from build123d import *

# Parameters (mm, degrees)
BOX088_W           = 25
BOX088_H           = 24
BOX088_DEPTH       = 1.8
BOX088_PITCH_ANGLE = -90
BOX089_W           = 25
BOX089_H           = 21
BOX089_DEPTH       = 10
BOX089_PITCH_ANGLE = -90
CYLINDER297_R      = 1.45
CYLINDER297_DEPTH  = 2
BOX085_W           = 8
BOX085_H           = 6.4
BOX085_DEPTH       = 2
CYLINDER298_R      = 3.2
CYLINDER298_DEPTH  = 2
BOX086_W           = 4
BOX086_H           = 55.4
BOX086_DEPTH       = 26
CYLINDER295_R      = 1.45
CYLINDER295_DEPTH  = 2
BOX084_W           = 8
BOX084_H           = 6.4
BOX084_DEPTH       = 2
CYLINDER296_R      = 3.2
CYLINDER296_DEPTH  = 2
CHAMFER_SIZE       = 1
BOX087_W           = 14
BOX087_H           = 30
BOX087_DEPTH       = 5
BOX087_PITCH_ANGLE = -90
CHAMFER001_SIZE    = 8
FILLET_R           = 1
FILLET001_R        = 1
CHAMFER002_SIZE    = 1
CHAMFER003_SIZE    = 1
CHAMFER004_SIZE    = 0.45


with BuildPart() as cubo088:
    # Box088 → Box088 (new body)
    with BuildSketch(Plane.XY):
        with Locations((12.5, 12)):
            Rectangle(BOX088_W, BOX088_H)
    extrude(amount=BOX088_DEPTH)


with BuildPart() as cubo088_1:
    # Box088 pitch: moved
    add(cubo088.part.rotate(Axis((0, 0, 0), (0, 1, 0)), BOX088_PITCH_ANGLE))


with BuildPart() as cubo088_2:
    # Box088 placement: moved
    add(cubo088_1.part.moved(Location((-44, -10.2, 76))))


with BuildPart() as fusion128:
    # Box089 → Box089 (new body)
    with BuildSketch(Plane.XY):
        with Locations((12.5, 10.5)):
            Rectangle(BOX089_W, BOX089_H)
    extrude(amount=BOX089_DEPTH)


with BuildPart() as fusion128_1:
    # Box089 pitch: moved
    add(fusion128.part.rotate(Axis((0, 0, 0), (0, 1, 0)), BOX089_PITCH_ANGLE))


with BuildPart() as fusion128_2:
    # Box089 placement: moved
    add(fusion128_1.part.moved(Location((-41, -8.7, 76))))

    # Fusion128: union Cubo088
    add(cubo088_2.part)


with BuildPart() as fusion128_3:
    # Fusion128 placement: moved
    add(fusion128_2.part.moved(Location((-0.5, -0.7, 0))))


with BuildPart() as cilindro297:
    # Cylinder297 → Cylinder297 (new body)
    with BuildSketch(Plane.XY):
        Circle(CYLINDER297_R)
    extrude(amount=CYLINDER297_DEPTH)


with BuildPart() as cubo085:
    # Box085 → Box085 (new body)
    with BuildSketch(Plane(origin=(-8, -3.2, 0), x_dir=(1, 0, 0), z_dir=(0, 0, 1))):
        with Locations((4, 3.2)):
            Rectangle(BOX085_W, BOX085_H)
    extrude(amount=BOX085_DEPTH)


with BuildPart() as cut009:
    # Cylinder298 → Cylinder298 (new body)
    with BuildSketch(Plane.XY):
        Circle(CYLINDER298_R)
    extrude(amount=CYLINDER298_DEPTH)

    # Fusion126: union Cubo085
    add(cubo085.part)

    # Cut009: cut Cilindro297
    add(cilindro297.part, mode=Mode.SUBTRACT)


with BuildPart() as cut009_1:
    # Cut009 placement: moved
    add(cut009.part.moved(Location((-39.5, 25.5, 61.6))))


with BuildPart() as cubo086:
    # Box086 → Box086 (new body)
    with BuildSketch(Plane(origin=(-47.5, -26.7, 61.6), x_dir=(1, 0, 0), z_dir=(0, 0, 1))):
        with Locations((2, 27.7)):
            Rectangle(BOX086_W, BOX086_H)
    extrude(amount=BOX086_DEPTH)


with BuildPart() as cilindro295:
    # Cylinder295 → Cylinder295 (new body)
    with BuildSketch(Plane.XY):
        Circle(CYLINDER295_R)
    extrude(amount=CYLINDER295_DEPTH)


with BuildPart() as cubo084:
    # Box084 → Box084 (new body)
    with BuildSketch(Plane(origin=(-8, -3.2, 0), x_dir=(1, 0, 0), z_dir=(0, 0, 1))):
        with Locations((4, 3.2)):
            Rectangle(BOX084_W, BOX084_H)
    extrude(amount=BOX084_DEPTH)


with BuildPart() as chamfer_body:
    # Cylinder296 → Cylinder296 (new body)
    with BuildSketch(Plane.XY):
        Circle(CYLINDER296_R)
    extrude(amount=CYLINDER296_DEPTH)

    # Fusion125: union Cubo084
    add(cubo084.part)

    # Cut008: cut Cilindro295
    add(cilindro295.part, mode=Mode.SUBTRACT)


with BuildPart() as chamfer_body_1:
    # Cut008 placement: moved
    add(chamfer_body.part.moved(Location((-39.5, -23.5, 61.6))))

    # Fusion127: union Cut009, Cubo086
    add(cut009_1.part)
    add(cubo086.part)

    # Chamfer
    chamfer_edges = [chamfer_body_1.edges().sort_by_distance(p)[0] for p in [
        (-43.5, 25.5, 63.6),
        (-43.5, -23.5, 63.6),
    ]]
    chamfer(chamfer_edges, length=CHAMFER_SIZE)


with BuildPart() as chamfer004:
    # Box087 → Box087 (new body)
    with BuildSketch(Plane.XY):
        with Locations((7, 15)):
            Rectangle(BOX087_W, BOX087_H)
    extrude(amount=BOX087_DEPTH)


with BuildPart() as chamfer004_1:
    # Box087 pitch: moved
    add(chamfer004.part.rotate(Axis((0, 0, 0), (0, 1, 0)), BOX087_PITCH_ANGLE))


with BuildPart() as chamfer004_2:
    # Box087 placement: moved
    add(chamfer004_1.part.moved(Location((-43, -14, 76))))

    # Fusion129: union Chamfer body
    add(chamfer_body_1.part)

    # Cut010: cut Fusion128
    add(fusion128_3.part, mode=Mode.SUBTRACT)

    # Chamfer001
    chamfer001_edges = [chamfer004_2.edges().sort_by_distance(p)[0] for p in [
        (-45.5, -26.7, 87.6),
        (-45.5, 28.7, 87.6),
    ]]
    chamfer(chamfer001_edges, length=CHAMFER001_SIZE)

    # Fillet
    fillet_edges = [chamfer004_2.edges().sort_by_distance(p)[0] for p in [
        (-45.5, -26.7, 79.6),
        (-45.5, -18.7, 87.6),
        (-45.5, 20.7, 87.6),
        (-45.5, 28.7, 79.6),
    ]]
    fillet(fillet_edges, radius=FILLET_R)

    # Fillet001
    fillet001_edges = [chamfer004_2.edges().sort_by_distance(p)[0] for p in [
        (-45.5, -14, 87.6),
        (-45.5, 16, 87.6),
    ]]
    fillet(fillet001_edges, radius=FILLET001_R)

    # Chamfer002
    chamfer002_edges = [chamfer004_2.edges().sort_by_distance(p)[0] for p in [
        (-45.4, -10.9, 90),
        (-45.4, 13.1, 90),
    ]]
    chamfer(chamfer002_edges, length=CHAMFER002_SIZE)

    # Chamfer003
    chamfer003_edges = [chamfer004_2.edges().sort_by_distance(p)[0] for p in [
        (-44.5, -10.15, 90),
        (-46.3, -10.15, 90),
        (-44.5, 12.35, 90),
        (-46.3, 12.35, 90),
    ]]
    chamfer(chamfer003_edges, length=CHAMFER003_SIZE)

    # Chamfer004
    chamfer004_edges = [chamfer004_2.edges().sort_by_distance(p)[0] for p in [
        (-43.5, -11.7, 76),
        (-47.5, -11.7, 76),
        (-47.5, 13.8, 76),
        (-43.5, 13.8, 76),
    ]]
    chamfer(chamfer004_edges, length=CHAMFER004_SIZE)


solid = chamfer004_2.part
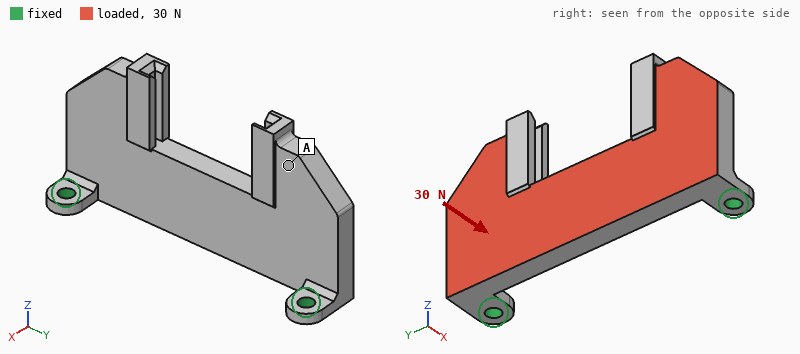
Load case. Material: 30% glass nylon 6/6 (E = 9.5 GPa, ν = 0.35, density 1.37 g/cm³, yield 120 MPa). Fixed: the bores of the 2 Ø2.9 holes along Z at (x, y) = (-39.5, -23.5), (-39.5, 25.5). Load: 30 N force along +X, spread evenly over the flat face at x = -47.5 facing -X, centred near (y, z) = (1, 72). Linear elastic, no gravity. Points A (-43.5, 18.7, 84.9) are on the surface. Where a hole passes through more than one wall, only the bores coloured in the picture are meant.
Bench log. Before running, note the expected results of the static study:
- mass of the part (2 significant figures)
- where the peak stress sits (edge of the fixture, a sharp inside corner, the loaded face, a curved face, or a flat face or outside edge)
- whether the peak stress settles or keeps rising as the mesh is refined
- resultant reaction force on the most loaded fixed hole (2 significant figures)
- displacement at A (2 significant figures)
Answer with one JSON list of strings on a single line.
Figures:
["6.6 g", "edge of the fixture", "keeps rising", "18 N", "0.25 mm"]
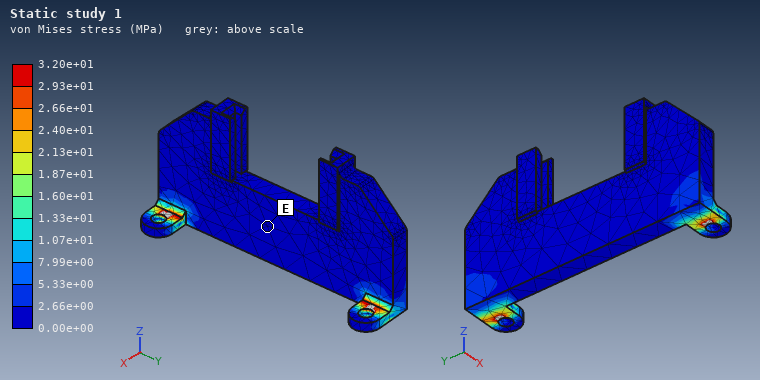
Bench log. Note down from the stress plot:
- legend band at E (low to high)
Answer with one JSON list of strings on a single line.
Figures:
["0.00e+00 to 2.66e+00 MPa"]
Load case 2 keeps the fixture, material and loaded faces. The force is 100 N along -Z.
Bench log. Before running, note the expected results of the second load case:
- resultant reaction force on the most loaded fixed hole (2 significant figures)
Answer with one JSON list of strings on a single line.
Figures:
["52 N"]
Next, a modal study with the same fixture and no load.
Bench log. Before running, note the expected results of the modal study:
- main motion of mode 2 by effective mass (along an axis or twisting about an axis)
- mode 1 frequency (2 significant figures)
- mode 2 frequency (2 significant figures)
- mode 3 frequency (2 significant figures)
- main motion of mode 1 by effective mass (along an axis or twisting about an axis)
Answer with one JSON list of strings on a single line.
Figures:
["twisting about Z", "740 Hz", "2000 Hz", "3700 Hz", "along X"]
